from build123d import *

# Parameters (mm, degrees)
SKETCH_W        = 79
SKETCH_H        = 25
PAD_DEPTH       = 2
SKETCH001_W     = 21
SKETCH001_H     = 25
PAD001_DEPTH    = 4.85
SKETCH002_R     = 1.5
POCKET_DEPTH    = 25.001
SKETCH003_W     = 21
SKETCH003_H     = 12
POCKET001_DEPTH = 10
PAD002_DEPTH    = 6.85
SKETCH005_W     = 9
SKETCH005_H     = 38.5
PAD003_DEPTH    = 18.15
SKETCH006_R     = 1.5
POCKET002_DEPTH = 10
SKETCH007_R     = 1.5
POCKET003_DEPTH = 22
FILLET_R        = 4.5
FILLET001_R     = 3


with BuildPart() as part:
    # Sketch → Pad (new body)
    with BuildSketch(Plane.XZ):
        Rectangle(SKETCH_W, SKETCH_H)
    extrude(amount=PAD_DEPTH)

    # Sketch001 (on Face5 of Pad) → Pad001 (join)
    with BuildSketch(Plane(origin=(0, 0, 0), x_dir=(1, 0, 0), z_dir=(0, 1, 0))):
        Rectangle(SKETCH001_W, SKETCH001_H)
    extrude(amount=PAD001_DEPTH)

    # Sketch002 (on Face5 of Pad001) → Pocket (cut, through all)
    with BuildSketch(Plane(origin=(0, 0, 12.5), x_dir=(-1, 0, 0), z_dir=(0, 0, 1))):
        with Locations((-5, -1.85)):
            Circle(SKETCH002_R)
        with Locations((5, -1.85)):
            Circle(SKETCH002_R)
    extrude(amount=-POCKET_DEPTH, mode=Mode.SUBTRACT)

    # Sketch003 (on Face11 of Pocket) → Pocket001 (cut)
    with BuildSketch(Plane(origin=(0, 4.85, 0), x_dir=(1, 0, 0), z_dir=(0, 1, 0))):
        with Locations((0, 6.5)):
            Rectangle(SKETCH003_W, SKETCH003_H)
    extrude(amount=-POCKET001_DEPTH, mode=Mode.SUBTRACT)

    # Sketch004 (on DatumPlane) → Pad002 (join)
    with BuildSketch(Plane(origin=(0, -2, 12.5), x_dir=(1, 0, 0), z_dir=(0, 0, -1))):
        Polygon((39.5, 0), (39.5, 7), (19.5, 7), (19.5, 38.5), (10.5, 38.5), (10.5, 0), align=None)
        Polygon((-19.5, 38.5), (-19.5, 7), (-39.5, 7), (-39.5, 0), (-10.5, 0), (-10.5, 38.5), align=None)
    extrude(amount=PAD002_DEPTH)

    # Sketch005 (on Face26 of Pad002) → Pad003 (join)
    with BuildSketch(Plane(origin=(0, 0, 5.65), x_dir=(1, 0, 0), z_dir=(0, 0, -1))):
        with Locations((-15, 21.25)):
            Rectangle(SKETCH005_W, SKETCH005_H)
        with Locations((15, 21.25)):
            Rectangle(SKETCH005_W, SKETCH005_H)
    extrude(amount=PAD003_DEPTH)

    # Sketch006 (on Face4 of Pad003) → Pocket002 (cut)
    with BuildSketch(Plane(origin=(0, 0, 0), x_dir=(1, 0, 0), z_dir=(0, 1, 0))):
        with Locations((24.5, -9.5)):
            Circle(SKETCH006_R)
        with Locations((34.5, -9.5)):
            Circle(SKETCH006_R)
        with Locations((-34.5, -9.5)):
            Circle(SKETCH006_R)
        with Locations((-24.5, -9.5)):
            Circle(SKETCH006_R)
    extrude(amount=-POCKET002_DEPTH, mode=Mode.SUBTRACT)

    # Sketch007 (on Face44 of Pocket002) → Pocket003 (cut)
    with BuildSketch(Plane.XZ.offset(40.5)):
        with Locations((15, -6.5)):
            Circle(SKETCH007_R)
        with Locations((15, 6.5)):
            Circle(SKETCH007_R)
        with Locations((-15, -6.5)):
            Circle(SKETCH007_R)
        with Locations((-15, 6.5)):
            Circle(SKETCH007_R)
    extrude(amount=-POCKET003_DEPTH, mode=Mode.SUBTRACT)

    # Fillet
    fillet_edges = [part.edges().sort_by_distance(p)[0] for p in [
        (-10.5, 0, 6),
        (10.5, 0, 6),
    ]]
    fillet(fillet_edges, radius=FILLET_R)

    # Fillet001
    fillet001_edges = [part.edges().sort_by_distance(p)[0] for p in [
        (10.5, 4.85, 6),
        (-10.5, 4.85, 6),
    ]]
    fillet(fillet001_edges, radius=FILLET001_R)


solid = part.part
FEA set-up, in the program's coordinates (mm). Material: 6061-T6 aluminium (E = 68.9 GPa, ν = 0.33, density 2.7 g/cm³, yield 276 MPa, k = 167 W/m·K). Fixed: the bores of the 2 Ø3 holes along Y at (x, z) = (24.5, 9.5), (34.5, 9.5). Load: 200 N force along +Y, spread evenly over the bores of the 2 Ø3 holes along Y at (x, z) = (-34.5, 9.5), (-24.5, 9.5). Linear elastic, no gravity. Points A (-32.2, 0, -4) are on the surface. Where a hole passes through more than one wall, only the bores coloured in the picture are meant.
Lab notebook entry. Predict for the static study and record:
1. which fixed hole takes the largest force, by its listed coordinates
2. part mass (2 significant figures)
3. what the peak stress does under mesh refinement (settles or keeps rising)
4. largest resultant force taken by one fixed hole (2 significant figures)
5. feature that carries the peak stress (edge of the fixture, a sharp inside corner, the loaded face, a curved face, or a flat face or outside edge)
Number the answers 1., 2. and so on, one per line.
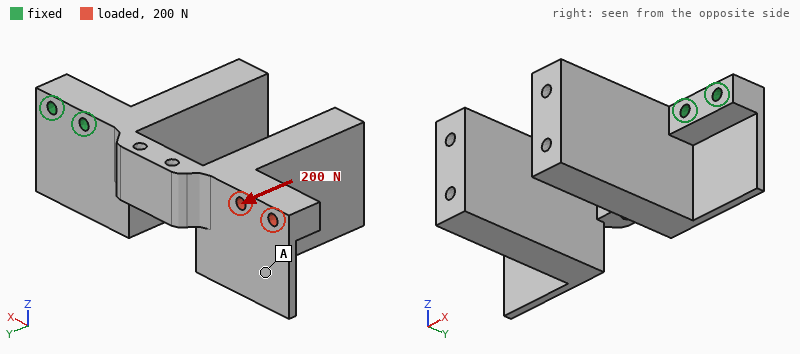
1. (24.5, 9.5)
2. 62 g
3. keeps rising
4. 320 N
5. a sharp inside corner
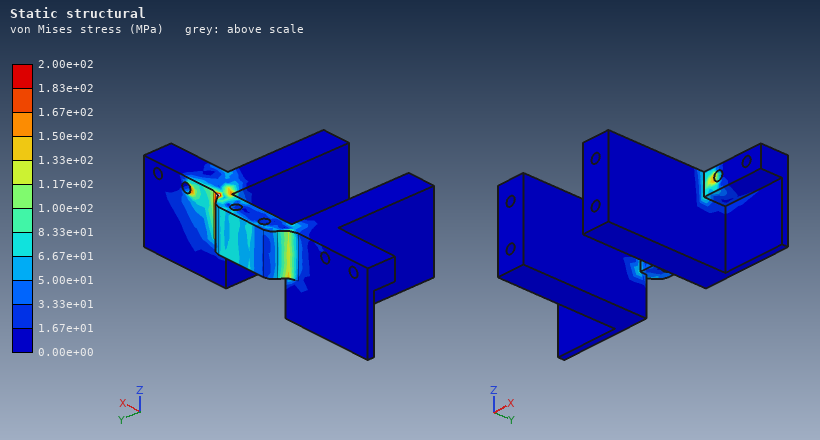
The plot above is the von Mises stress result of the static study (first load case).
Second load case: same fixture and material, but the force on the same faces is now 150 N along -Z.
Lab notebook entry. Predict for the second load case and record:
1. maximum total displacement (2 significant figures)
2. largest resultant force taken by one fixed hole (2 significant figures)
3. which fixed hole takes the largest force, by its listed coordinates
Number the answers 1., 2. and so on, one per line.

1. 0.21 mm
2. 680 N
3. (24.5, 9.5)
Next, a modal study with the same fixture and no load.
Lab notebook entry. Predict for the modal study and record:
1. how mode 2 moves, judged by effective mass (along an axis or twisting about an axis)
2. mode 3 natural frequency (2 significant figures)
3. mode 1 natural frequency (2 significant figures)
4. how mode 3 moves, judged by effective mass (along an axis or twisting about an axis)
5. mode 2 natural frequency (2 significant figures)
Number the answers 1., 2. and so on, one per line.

1. along Z
2. 1700 Hz
3. 560 Hz
4. along Y
5. 800 Hz
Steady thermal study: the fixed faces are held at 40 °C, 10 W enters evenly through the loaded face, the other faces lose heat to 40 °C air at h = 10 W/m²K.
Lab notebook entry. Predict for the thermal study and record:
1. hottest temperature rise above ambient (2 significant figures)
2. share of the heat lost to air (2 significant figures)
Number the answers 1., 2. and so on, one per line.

1. 39 K
2. 19 %
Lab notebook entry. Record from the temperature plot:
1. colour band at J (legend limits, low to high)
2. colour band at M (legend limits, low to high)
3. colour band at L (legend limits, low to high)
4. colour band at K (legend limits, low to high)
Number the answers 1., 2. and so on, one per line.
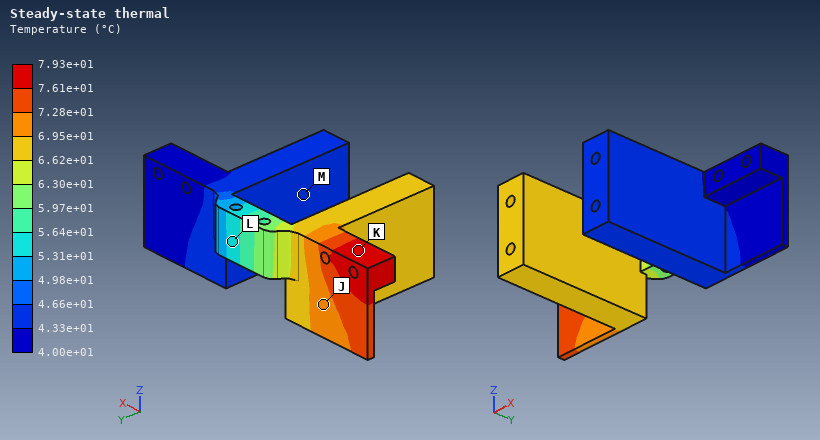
1. 6.95e+01 to 7.28e+01 °C
2. 4.33e+01 to 4.66e+01 °C
3. 5.31e+01 to 5.64e+01 °C
4. 7.61e+01 to 7.93e+01 °C
